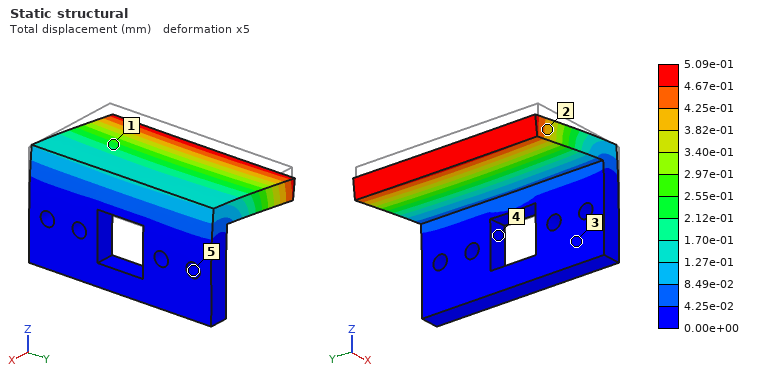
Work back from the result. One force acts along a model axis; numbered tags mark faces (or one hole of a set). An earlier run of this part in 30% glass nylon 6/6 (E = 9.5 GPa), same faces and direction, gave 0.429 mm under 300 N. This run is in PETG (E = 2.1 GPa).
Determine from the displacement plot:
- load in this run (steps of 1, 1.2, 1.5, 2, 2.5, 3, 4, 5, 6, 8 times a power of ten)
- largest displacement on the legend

80 N
5.09e-01 mm
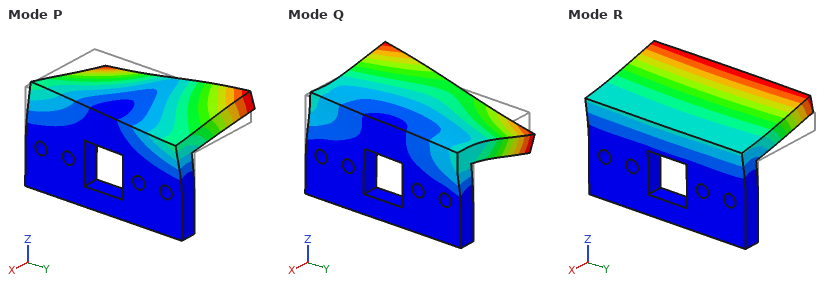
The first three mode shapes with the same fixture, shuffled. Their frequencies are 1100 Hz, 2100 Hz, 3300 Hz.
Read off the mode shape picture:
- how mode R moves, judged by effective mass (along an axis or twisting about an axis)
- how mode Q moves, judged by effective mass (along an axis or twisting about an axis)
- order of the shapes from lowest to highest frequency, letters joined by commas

along Z
along Y
R, P, Q
